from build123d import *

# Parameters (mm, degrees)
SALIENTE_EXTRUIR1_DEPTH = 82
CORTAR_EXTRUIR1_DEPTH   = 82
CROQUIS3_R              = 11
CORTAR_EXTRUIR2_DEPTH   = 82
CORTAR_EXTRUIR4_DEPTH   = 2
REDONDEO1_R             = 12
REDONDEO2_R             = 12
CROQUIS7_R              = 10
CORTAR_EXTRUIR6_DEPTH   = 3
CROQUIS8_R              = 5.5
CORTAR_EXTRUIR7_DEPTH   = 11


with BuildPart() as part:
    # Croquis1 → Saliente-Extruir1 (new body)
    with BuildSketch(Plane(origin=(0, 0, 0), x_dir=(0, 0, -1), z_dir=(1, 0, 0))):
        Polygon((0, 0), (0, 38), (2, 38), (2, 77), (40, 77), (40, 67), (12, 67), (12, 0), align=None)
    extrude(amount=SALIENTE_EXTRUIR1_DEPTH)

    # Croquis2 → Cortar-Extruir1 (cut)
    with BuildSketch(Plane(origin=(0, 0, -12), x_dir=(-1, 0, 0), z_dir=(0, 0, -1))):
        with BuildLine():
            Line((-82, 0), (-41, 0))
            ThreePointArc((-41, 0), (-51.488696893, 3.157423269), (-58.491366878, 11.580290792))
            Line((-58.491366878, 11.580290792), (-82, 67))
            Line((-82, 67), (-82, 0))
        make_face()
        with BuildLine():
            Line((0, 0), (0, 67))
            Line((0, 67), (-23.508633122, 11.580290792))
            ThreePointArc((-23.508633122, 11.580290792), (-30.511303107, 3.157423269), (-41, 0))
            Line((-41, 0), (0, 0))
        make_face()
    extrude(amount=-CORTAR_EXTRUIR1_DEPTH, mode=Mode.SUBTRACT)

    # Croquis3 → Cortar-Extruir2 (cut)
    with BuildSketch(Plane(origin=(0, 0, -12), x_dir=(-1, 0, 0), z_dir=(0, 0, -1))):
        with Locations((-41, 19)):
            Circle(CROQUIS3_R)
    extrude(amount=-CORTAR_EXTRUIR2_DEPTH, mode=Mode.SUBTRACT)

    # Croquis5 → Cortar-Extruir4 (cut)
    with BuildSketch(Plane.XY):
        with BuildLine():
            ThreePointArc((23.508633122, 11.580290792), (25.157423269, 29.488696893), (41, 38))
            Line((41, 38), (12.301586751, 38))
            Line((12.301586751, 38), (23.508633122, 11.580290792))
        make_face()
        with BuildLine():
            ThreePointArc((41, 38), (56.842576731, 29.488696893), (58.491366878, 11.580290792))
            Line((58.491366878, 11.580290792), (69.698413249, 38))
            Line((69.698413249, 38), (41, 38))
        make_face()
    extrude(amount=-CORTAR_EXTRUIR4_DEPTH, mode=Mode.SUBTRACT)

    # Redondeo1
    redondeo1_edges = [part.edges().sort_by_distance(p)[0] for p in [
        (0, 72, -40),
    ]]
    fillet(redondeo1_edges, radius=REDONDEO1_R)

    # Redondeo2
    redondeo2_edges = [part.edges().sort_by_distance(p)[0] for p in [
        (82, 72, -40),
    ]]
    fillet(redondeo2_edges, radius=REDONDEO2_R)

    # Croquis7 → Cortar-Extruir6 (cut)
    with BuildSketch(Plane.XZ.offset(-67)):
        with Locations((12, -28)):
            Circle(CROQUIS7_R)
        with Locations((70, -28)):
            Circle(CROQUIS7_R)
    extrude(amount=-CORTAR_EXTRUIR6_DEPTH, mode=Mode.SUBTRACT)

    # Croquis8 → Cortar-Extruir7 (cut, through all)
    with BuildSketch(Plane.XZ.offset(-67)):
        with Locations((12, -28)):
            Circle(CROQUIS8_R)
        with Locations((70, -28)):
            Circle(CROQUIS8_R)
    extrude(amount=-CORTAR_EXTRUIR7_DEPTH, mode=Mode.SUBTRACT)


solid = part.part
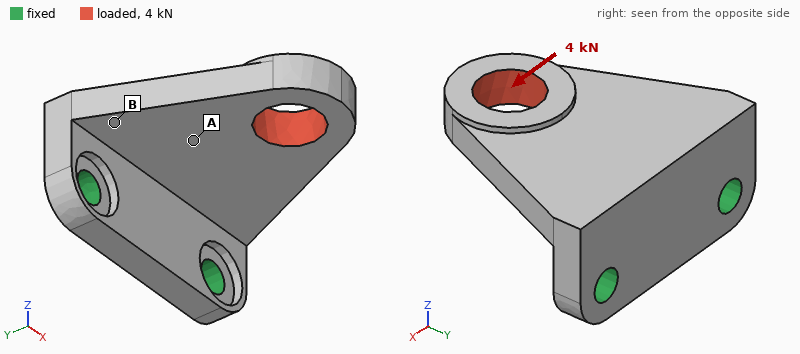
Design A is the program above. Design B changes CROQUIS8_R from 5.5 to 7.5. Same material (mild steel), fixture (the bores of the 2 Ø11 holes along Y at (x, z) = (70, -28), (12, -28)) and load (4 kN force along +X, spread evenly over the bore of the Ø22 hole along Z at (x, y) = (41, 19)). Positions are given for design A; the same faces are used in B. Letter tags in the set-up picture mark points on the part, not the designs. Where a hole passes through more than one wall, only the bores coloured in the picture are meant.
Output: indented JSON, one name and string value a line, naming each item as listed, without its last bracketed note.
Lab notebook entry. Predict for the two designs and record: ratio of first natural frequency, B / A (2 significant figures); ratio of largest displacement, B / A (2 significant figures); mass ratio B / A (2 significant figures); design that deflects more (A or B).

{
  "ratio of first natural frequency, B / A": "1.1",
  "ratio of largest displacement, B / A": "0.81",
  "mass ratio B / A": "0.98",
  "design that deflects more": "A"
}
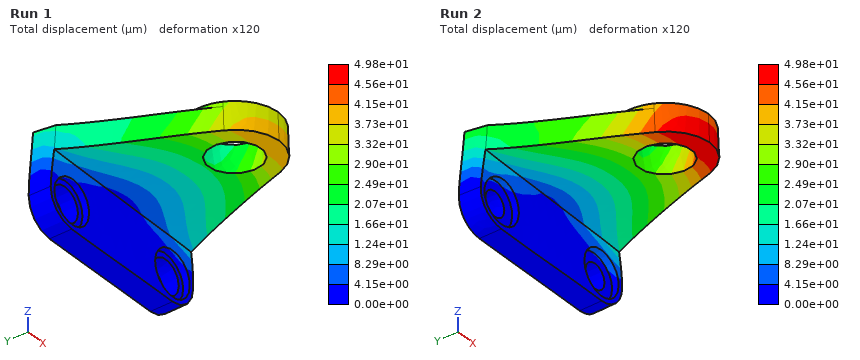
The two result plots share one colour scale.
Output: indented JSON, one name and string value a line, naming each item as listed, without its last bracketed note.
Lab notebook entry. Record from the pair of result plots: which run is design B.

{
  "which run is design B": "Run 1"
}
